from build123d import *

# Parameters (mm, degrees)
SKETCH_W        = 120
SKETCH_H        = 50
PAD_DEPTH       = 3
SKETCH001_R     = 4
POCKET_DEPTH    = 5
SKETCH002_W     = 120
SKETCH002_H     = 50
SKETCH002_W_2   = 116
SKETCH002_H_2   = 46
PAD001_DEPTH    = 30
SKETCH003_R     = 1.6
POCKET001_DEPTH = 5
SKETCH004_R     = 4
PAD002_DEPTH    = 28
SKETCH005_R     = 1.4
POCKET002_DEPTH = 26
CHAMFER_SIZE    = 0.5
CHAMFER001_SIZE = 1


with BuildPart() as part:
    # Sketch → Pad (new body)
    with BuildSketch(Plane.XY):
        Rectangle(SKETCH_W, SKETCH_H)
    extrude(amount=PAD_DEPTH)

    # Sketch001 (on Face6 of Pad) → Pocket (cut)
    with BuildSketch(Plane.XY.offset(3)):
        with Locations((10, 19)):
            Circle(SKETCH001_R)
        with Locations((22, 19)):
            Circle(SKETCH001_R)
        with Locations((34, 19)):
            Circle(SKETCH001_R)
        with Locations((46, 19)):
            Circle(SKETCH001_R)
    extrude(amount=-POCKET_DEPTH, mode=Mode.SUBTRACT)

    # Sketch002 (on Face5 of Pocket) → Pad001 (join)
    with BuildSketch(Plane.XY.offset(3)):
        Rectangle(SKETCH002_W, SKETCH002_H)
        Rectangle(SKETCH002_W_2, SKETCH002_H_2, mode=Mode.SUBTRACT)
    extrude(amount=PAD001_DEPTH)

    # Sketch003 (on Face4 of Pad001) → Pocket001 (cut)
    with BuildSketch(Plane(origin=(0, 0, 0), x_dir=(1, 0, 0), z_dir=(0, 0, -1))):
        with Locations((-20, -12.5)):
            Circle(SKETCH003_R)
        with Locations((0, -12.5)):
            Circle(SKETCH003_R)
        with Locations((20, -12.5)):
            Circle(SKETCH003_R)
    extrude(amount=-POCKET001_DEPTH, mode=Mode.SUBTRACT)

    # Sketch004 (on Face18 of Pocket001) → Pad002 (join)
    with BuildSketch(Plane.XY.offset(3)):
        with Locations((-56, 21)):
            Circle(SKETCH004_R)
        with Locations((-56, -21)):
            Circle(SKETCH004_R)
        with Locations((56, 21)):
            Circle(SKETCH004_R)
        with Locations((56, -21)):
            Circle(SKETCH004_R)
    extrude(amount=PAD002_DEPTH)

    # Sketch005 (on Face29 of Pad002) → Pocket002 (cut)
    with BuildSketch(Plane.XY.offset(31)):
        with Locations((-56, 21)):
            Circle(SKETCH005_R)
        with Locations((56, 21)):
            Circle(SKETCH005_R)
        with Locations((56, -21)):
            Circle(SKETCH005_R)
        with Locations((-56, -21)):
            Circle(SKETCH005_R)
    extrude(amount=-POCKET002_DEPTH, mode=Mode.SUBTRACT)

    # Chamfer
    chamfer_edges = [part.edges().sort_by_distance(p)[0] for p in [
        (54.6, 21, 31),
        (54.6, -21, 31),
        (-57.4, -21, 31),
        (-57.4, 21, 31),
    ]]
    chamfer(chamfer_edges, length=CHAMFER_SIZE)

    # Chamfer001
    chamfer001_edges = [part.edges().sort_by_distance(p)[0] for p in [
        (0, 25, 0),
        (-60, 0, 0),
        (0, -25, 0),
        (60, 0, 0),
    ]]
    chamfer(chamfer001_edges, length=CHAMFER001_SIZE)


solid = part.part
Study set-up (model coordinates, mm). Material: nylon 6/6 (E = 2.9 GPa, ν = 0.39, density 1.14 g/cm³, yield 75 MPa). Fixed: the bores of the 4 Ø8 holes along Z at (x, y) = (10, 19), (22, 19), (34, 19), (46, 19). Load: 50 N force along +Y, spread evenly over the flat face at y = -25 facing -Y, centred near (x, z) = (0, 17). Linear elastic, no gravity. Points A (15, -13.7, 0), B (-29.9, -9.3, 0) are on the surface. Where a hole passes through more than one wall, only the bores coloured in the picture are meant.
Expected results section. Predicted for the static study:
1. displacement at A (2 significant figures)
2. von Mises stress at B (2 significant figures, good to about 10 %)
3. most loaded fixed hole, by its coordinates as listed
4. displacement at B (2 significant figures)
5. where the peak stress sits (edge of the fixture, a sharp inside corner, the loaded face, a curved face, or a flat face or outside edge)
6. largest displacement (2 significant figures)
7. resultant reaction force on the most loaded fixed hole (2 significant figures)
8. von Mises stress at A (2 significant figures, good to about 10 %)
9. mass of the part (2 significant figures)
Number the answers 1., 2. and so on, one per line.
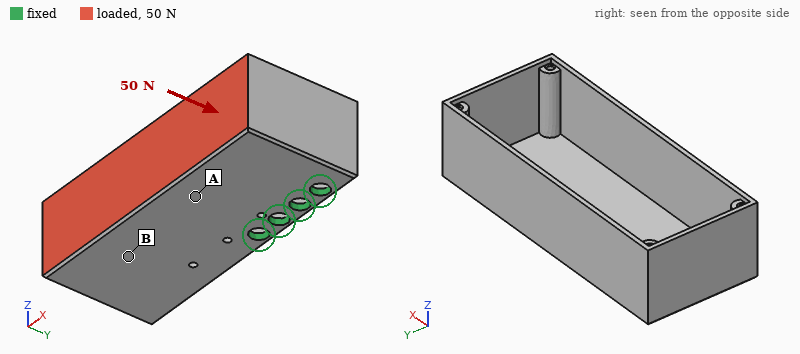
1. 0.32 mm
2. 1.3 MPa
3. (10, 19)
4. 0.56 mm
5. a flat face or outside edge
6. 1.5 mm
7. 59 N
8. 2.4 MPa
9. 46 g
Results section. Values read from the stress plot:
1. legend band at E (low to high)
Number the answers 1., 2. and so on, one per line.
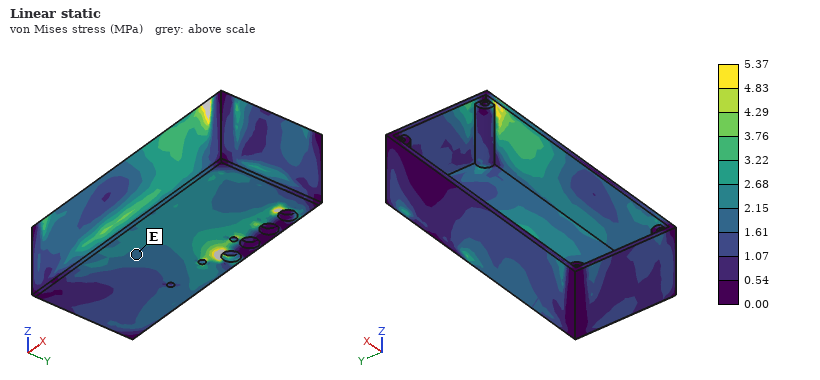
1. 1.61 to 2.15 MPa
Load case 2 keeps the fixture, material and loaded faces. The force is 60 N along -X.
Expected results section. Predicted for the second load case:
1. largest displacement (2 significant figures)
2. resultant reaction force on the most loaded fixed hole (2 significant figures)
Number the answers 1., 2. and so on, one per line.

1. 1.3 mm
2. 61 N
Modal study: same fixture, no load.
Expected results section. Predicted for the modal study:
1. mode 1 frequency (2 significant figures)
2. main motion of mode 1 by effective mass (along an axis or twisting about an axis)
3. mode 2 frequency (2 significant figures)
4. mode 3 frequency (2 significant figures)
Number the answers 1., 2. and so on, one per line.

1. 150 Hz
2. along Z
3. 400 Hz
4. 580 Hz
